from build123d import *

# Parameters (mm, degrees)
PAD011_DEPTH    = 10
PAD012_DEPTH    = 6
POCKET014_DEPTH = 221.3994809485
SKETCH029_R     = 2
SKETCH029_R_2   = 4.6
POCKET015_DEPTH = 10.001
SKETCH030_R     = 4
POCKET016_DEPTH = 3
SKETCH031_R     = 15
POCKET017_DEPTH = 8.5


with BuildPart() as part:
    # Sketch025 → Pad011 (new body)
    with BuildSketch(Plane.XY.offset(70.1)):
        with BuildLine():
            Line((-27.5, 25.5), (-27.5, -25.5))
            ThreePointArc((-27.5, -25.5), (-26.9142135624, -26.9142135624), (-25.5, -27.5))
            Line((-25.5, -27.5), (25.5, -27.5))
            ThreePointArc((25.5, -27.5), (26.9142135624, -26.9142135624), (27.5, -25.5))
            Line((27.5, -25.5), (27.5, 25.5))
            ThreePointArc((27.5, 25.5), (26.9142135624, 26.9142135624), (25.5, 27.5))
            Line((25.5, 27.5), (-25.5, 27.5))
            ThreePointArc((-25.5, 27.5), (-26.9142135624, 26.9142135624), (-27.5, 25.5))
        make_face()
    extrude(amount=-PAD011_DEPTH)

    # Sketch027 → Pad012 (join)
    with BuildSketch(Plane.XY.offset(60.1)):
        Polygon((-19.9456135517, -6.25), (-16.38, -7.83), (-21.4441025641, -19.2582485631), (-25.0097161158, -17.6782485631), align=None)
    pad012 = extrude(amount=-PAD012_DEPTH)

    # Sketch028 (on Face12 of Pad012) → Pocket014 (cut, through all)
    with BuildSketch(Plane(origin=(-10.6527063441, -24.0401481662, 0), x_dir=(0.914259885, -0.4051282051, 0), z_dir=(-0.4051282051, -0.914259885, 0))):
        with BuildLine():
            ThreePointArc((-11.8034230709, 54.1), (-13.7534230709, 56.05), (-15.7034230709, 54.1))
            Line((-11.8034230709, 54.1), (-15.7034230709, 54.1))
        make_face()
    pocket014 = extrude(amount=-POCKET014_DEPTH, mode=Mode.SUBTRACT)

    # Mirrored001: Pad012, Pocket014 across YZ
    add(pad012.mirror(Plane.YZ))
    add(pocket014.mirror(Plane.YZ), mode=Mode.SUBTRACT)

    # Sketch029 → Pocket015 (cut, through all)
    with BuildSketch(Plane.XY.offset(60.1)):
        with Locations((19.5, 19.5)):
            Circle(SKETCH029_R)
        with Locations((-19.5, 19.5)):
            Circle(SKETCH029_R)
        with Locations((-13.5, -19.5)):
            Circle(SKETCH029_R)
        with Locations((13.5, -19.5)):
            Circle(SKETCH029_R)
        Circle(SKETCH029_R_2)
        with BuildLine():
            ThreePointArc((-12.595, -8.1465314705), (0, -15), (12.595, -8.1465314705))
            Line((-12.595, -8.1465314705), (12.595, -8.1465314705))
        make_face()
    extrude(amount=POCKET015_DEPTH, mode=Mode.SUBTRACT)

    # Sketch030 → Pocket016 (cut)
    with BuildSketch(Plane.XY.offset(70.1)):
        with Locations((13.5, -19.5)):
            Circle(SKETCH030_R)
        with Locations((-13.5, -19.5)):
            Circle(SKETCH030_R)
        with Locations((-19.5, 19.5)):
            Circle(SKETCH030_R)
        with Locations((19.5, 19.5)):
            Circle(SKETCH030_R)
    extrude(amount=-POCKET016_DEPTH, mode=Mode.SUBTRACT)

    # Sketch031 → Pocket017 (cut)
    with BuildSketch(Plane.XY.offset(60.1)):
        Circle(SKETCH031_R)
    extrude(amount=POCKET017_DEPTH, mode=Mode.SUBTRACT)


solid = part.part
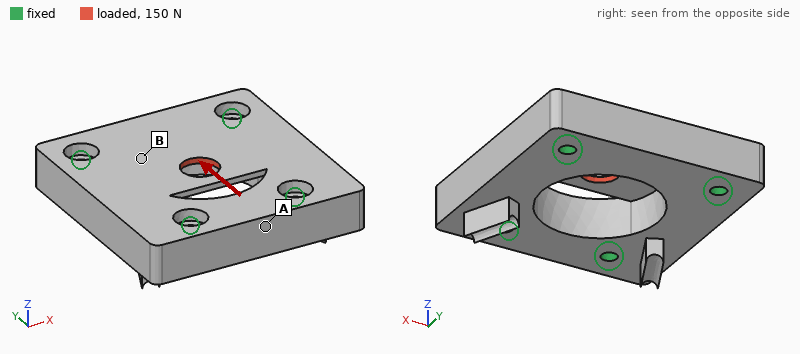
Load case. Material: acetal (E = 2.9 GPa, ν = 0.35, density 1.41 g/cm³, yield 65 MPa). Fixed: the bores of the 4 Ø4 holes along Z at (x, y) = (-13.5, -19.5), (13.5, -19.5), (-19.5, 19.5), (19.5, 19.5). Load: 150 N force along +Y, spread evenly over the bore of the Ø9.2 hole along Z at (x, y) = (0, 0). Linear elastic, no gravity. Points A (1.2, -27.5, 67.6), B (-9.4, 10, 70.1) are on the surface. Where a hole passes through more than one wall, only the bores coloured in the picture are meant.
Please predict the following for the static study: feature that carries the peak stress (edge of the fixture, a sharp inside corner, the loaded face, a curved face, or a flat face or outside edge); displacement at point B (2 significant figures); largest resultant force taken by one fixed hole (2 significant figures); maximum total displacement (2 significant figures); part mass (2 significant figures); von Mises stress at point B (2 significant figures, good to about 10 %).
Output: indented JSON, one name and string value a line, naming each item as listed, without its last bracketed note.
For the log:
{
  "feature that carries the peak stress": "a flat face or outside edge",
  "displacement at point B": "12 µm",
  "largest resultant force taken by one fixed hole": "58 N",
  "maximum total displacement": "49 µm",
  "part mass": "33 g",
  "von Mises stress at point B": "2.3 MPa"
}
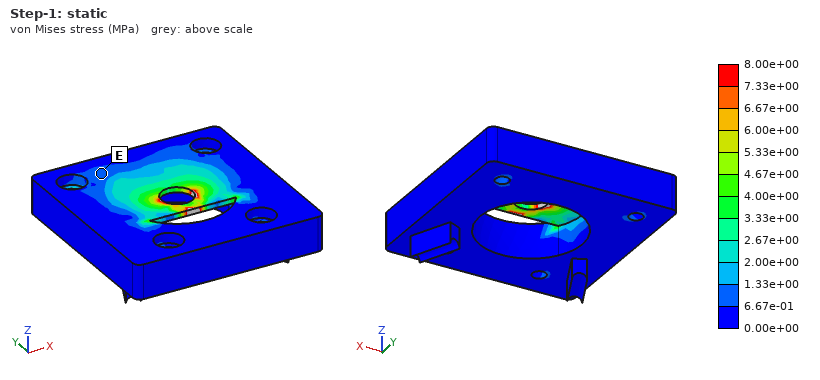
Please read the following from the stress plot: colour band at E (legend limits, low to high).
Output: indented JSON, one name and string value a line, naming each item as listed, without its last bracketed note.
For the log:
{
  "colour band at E": "6.67e-01 to 1.33e+00 MPa"
}
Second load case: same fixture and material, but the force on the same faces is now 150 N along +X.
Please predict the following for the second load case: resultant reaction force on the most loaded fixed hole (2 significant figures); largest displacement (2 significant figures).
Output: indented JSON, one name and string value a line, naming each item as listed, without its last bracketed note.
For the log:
{
  "resultant reaction force on the most loaded fixed hole": "47 N",
  "largest displacement": "25 µm"
}
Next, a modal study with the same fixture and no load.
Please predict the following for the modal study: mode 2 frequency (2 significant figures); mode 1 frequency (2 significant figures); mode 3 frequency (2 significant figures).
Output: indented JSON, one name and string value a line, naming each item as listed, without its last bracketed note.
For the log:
{
  "mode 2 frequency": "5000 Hz",
  "mode 1 frequency": "3300 Hz",
  "mode 3 frequency": "5200 Hz"
}
